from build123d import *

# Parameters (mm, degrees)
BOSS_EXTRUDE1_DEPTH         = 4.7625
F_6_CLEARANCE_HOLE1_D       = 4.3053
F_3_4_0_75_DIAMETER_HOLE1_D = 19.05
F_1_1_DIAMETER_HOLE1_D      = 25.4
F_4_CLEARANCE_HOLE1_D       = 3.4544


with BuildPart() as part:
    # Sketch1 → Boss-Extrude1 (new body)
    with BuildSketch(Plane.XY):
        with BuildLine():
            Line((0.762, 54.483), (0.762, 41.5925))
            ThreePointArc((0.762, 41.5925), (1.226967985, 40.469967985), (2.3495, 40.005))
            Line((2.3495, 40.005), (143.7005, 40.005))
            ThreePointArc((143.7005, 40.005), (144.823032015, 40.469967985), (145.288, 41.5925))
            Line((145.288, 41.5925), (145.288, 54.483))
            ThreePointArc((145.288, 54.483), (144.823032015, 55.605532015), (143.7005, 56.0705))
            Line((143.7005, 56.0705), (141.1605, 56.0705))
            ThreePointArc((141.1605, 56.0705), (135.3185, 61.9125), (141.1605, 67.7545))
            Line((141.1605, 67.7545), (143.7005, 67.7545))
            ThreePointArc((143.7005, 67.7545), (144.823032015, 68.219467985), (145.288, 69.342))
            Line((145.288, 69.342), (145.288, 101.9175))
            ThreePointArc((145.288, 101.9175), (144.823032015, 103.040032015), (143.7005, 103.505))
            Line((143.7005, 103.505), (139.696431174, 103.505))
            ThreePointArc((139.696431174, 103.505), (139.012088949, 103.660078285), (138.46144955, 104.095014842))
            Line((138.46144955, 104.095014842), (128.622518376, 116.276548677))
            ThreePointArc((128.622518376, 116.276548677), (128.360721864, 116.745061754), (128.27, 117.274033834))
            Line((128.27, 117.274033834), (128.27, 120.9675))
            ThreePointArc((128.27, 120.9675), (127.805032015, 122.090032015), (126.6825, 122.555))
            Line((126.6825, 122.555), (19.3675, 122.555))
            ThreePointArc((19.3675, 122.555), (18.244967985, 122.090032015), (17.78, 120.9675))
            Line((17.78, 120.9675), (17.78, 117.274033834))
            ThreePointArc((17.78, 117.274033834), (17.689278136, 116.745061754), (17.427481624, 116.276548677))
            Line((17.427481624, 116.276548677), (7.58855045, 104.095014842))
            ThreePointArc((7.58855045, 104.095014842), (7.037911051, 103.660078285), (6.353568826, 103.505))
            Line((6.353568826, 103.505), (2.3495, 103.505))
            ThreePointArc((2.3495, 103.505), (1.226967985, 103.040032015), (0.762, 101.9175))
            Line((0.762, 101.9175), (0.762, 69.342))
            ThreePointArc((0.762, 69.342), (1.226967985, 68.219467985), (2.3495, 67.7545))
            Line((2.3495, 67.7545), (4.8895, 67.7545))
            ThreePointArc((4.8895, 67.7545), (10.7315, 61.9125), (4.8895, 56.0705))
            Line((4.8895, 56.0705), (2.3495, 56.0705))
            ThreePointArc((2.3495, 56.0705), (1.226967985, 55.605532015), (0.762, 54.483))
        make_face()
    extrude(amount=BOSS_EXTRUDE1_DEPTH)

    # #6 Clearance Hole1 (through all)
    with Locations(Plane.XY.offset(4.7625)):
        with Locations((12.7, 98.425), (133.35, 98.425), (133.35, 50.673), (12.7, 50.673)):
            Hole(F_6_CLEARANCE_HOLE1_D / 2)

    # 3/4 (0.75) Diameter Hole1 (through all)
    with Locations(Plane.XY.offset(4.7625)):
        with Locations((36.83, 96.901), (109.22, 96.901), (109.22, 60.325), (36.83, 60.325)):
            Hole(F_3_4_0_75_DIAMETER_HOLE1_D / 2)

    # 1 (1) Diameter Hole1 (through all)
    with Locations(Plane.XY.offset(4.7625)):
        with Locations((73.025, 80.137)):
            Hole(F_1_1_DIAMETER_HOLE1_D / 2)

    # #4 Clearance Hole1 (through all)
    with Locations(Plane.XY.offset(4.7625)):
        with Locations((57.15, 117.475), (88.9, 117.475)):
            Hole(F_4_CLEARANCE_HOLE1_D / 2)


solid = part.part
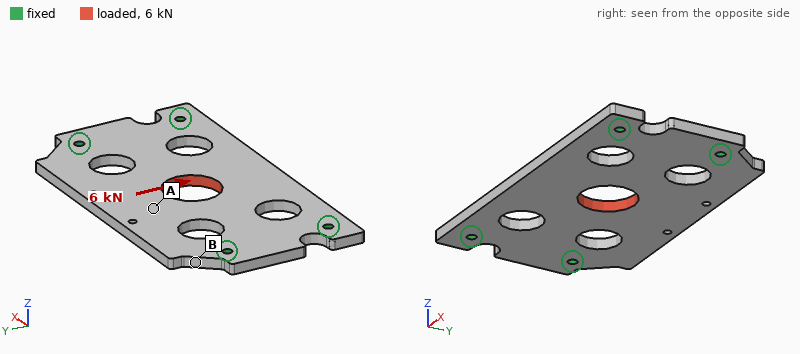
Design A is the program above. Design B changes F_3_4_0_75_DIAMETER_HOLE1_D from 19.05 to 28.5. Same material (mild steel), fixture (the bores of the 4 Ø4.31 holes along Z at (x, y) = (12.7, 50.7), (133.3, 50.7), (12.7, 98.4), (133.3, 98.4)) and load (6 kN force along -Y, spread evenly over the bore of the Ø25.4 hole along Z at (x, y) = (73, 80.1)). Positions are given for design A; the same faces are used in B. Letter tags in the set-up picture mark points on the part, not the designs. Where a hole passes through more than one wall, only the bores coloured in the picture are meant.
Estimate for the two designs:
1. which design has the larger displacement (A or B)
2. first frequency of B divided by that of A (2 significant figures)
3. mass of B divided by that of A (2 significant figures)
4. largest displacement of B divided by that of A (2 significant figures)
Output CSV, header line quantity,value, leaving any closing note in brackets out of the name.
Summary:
quantity,value
which design has the larger displacement,B
first frequency of B divided by that of A,0.93
mass of B divided by that of A,0.85
largest displacement of B divided by that of A,2.3
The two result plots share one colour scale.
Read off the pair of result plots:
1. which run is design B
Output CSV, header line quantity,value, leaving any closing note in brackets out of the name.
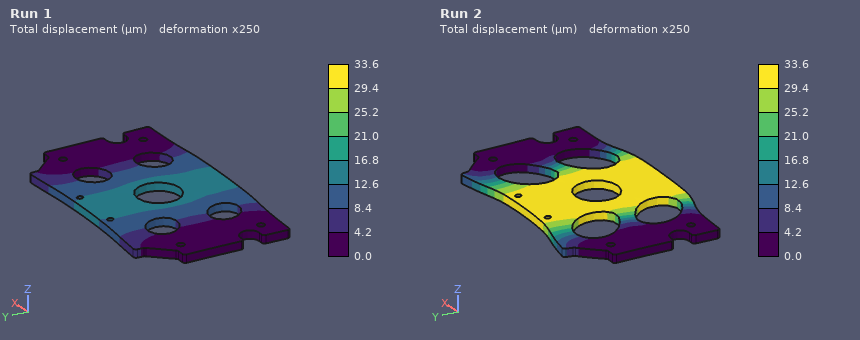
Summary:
quantity,value
which run is design B,Run 2
